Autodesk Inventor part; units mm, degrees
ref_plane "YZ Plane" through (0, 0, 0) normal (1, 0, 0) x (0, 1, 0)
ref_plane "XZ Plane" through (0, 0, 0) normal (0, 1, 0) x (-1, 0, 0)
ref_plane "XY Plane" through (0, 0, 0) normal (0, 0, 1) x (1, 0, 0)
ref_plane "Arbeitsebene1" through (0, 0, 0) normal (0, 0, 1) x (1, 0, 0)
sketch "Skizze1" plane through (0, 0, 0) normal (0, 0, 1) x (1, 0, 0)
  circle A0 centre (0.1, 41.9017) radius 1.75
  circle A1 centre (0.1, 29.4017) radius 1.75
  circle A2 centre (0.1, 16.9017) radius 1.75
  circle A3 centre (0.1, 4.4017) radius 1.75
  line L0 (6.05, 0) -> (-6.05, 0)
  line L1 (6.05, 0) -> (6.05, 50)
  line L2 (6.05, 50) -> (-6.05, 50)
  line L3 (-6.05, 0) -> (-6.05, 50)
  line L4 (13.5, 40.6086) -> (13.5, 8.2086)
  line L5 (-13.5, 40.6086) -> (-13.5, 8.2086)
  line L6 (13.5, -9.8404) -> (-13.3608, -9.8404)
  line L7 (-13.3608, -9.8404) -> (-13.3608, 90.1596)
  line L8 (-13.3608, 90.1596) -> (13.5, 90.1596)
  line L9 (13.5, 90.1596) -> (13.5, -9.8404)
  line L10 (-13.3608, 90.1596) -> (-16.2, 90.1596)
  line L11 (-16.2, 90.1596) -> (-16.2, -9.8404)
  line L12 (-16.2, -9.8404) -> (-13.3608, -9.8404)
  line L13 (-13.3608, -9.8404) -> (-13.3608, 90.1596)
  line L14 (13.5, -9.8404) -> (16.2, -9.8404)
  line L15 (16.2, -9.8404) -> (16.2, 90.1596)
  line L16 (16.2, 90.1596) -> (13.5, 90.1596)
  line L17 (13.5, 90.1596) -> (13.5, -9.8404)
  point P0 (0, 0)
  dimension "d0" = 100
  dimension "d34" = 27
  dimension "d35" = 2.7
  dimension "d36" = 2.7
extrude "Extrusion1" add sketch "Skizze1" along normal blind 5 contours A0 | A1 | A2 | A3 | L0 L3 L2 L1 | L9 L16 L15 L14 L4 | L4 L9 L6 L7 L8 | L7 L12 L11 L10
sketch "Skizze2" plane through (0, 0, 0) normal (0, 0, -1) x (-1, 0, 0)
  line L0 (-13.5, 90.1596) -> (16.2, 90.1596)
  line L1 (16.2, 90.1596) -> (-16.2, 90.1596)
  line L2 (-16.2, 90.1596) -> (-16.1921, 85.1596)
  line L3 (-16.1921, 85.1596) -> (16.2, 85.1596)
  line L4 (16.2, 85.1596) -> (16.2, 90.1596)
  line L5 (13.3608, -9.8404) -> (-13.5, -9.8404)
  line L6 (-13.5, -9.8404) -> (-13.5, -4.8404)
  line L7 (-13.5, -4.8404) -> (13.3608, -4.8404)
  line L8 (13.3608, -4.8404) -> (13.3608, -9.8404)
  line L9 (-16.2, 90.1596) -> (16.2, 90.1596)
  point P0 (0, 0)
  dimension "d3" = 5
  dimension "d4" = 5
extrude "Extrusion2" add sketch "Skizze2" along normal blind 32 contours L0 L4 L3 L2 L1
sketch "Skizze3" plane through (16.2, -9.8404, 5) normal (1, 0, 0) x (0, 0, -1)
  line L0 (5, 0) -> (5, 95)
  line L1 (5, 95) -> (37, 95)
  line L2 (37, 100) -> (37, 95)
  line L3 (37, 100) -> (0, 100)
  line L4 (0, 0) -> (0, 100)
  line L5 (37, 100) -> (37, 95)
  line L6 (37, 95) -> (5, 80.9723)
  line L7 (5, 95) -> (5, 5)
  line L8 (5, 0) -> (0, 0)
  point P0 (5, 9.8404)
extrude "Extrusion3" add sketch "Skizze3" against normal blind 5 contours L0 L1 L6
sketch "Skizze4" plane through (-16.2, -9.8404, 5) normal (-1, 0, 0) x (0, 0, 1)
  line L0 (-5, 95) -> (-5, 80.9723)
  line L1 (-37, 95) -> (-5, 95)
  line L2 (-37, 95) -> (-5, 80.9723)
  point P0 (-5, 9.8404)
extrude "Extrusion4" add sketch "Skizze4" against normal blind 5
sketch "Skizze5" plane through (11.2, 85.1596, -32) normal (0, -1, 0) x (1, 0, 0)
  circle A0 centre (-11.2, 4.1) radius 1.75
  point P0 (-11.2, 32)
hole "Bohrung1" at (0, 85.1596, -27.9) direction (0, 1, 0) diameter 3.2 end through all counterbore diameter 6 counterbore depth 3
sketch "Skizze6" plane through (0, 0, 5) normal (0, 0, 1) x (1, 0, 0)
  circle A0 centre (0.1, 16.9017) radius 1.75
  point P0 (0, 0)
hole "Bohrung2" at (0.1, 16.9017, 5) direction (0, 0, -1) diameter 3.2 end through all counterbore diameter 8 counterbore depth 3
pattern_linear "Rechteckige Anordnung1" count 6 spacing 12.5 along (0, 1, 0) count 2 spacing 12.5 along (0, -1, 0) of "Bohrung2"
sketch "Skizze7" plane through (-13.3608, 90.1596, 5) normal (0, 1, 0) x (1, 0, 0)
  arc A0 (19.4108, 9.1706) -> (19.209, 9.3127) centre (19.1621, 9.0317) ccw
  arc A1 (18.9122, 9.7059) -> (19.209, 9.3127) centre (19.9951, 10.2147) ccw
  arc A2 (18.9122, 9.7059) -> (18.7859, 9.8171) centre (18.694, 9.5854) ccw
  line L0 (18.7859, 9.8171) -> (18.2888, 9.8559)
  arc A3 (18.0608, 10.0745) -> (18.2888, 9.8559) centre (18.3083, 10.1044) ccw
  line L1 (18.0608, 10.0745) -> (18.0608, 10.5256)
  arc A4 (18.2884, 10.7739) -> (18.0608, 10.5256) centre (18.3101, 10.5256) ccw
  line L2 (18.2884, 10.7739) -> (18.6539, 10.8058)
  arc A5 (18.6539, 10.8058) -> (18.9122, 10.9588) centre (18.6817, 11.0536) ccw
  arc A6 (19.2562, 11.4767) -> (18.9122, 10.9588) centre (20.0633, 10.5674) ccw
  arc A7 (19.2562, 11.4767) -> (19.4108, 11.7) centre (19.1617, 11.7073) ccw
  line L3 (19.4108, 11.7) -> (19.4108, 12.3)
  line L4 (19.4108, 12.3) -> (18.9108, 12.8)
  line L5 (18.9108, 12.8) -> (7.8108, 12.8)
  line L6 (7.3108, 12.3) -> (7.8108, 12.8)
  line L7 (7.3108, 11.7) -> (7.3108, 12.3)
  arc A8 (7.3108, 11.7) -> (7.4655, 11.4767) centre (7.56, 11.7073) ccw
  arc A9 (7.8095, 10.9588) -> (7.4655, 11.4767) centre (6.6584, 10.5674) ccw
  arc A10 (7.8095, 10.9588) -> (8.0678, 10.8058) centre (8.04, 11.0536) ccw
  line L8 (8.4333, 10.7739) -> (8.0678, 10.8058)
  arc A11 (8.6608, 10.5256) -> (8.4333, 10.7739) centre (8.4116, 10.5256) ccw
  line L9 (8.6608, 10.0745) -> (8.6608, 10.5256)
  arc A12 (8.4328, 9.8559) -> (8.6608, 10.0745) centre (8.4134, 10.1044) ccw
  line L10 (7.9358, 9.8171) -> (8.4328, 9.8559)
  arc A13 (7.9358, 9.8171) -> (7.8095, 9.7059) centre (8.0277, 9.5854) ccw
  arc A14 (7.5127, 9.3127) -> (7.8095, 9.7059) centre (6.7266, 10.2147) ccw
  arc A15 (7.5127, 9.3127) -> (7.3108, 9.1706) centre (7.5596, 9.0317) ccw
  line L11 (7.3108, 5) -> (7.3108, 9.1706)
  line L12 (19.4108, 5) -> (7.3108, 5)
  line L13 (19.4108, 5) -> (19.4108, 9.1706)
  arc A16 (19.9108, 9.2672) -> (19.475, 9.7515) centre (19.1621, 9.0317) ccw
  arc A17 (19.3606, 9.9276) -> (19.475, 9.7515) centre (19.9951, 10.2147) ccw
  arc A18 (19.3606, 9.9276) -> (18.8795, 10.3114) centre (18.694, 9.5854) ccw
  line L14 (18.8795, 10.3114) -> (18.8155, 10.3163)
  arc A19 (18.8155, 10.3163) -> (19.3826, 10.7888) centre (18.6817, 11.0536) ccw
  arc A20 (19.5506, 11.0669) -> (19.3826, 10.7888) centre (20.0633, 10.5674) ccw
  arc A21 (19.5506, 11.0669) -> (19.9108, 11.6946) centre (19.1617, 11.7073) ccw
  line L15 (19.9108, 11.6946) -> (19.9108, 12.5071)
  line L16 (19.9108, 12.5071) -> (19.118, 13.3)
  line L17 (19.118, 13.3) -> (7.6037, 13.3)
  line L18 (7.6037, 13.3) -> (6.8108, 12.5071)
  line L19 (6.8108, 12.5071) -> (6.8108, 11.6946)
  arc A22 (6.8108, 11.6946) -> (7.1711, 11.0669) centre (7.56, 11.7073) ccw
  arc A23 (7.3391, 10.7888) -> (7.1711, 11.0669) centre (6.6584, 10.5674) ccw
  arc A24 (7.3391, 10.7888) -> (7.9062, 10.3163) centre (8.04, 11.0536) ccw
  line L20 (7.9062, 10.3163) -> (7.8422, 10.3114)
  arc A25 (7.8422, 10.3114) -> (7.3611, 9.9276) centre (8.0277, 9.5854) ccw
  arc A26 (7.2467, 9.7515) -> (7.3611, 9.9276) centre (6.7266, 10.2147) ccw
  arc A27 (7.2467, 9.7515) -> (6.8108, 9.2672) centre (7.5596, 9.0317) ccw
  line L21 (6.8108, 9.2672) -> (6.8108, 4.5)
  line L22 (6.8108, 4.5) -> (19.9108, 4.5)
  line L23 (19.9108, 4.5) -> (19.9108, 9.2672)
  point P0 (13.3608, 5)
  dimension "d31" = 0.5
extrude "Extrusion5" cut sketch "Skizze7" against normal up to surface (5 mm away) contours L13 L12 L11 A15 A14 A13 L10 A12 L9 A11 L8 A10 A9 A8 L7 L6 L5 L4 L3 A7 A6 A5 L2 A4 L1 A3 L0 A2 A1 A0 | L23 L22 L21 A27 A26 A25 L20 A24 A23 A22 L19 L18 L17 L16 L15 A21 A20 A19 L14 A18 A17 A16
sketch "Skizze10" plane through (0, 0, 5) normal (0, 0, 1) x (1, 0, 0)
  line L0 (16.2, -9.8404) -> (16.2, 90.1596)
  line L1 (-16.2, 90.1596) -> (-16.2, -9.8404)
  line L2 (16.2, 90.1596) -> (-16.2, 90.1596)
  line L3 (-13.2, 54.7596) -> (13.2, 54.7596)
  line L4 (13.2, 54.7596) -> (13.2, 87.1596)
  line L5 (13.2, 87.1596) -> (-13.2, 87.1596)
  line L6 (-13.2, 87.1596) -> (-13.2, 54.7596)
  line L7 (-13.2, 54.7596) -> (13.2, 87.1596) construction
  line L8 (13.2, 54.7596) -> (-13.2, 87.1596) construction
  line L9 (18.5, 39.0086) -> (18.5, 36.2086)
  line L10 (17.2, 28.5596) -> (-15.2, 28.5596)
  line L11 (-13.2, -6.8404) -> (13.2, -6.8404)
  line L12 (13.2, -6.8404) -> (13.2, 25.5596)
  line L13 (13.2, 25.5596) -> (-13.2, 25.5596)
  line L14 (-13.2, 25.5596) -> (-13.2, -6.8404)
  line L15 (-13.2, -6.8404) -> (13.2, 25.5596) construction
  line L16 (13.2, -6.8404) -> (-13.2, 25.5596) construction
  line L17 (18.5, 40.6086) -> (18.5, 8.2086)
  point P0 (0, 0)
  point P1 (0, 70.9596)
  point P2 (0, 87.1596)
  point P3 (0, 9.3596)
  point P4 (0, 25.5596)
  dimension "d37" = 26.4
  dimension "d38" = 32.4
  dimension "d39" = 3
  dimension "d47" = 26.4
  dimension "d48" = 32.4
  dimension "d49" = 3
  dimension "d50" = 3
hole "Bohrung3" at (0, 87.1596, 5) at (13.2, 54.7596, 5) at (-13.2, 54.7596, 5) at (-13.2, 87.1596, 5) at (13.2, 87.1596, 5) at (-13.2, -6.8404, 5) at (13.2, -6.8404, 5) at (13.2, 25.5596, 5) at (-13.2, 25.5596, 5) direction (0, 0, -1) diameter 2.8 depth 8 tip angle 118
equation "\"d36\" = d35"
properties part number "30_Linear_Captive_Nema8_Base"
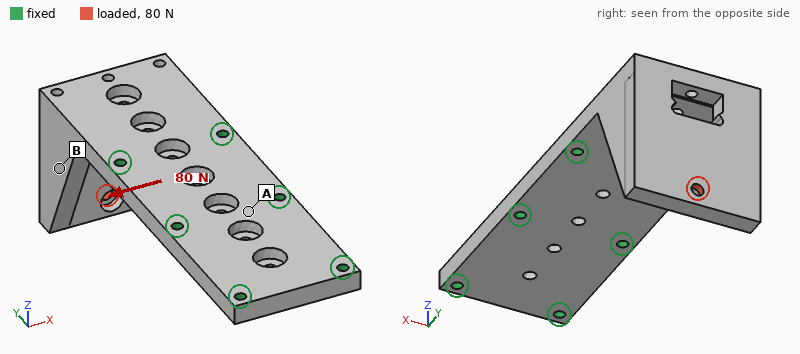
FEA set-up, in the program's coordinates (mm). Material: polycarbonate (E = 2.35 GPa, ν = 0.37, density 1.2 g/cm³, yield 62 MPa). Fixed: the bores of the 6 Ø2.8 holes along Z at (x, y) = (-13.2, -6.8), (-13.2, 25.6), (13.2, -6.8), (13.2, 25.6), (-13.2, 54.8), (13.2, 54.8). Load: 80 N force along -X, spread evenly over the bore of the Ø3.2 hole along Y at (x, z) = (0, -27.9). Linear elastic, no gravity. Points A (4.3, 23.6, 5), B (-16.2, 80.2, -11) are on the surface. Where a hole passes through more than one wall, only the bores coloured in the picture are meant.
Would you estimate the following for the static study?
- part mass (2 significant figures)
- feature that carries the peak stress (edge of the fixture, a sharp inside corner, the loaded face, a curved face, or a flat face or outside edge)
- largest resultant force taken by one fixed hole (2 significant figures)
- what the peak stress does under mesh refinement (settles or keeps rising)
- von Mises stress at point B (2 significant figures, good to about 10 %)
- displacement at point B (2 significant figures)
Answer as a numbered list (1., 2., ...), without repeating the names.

1. 26 g
2. edge of the fixture
3. 140 N
4. keeps rising
5. 2.9 MPa
6. 0.61 mm
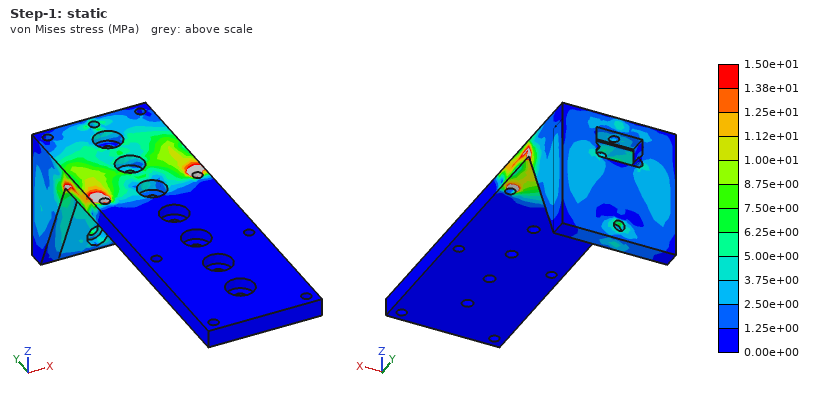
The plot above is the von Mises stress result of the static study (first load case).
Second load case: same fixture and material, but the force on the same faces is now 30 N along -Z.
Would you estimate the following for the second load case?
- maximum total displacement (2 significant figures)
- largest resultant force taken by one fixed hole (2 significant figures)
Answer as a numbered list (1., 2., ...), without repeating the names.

1. 1.0 mm
2. 20 N
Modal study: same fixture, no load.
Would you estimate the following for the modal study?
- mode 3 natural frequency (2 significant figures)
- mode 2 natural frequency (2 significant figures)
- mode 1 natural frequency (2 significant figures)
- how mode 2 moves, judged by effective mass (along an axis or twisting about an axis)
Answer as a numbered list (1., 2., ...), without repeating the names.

1. 1600 Hz
2. 680 Hz
3. 320 Hz
4. along X
